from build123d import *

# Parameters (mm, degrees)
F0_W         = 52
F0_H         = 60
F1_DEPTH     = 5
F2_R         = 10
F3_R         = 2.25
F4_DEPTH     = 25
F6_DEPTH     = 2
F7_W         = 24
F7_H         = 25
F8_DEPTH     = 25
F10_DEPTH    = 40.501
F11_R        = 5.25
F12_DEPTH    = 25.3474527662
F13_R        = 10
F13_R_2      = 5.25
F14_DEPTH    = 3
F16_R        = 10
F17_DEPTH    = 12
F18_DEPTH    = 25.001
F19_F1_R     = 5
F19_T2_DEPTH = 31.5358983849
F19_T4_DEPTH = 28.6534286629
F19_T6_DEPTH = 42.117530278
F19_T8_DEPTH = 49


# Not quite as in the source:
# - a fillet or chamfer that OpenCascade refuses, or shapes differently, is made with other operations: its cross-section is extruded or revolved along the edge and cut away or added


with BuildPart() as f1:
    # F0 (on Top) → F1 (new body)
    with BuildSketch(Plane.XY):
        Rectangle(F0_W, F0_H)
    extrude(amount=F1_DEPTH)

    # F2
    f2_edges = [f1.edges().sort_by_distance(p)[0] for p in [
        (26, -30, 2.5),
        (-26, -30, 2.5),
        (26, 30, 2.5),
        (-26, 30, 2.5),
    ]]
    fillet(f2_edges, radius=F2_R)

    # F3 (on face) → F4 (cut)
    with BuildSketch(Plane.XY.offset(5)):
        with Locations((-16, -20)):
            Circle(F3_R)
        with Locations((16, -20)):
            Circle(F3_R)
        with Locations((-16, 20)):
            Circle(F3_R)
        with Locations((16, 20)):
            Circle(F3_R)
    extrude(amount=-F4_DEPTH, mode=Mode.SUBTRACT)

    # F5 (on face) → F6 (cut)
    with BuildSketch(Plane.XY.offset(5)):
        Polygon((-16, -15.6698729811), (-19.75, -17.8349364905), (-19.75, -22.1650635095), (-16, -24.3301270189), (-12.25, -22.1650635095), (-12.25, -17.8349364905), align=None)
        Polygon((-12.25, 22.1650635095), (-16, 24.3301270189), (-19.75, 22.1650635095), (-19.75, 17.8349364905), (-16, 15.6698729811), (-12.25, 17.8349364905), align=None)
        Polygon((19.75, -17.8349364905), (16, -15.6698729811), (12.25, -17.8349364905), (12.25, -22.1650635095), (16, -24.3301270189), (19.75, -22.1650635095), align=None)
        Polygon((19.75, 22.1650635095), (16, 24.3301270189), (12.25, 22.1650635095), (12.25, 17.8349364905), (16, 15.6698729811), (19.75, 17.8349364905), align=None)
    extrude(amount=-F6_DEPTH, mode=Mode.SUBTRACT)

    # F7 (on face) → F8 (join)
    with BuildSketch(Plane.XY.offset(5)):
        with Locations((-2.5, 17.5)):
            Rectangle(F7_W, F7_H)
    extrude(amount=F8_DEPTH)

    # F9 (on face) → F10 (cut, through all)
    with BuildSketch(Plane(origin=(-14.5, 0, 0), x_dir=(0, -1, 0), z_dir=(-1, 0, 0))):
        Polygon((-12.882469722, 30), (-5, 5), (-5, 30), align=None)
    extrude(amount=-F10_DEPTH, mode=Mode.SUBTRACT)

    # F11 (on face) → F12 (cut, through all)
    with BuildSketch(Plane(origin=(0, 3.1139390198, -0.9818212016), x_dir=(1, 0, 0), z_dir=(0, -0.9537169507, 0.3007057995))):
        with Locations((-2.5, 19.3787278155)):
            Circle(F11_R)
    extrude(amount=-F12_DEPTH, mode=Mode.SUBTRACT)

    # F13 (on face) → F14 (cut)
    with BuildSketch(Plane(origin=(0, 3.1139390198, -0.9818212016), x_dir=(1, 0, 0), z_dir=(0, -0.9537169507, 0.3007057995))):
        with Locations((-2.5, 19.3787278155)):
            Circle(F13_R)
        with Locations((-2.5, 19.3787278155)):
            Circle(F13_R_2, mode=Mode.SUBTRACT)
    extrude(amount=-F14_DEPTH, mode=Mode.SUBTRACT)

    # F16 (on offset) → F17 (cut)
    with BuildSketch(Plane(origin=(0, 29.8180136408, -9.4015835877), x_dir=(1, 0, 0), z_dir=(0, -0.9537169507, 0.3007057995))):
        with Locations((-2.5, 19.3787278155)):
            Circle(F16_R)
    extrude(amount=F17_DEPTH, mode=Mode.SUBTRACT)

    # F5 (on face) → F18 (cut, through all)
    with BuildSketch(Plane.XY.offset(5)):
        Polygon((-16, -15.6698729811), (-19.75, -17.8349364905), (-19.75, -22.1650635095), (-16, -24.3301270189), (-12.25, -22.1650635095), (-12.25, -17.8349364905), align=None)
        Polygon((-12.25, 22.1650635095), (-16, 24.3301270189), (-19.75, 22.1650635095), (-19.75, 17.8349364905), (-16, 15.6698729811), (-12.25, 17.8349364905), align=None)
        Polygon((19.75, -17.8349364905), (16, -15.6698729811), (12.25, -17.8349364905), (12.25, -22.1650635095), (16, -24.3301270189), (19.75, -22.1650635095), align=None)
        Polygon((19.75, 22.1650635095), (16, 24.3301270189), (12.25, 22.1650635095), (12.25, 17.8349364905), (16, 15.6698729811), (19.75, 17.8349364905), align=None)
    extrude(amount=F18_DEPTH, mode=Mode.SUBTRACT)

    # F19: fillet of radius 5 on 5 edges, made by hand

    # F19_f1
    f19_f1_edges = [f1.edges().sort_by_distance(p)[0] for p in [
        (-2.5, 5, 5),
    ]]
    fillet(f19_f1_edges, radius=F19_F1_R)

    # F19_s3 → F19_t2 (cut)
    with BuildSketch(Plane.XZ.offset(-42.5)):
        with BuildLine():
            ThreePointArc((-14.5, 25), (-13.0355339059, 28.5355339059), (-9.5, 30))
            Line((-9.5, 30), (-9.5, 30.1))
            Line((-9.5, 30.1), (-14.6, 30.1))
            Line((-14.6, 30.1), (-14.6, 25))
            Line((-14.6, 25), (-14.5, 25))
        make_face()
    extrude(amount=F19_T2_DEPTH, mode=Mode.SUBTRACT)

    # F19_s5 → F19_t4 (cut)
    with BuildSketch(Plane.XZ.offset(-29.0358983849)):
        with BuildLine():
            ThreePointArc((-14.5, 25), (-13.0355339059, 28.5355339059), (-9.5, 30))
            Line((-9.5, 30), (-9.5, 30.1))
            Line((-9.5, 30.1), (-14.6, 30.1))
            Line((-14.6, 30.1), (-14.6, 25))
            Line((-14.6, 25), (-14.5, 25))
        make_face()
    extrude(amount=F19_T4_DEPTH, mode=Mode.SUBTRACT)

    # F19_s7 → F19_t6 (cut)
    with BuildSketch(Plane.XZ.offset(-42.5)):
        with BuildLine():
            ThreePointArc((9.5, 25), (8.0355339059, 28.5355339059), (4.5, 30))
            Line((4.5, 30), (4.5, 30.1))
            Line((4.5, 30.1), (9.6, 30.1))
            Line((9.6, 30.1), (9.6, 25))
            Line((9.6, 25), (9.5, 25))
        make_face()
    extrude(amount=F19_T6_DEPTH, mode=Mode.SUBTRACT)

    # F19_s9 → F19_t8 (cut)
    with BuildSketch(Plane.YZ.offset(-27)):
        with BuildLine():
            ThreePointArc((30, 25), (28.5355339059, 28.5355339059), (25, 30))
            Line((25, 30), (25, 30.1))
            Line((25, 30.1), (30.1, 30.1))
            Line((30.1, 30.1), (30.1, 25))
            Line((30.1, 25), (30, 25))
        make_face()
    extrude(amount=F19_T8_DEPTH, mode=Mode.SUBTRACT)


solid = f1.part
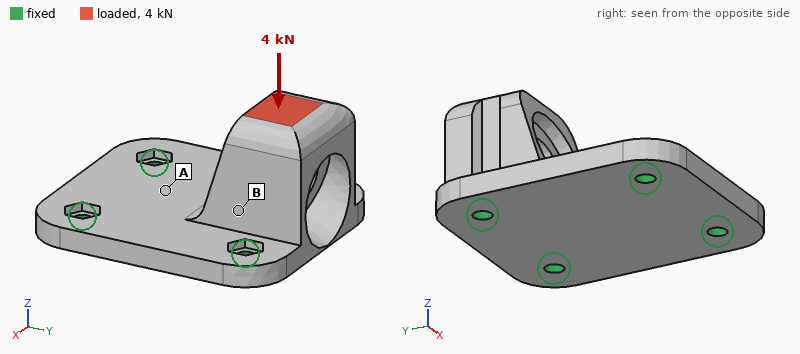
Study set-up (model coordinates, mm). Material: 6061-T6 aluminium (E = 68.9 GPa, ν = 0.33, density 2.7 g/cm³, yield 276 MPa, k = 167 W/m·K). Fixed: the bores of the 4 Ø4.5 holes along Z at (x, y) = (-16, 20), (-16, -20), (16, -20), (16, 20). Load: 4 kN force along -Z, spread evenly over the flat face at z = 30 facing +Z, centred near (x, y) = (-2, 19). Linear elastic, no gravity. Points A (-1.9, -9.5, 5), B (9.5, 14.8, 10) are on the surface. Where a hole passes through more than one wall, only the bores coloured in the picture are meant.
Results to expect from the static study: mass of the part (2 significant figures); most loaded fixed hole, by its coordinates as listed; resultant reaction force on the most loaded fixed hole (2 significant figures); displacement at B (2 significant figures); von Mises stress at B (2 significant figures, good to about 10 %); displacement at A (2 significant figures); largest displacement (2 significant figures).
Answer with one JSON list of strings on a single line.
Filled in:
["61 g", "(-16, 20)", "2.4 kN", "17 µm", "26 MPa", "5.8 µm", "25 µm"]
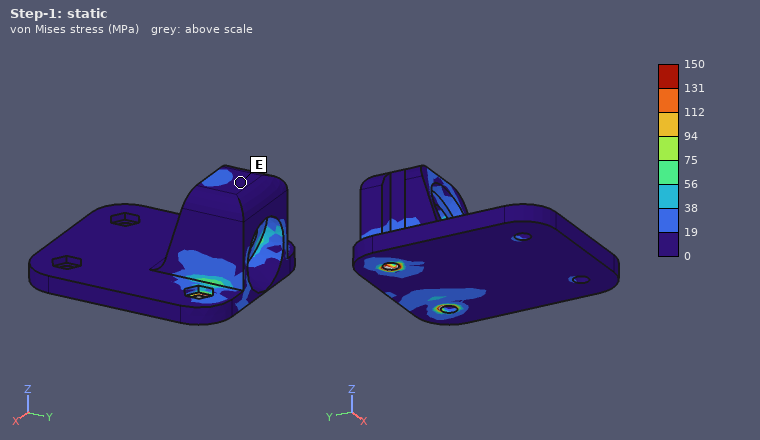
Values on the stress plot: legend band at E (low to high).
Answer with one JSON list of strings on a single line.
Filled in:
["0 to 19 MPa"]
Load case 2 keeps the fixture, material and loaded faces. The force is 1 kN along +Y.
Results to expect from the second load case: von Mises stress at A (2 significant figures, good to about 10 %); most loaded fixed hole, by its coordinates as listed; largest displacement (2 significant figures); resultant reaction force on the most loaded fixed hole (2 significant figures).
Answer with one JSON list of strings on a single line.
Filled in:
["14 MPa", "(-16, -20)", "67 µm", "760 N"]
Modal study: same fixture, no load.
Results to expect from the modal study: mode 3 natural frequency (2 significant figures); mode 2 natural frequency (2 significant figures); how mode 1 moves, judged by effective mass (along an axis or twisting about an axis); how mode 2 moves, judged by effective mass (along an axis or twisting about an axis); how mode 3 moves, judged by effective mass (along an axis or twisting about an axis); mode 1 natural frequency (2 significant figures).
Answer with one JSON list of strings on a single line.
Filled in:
["13 kHz", "9800 Hz", "along Y", "along X", "along Z", "6100 Hz"]
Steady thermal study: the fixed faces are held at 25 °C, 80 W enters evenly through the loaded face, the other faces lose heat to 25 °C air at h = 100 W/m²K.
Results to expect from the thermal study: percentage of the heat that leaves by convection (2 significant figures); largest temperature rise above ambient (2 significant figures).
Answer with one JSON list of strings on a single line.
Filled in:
["19 %", "64 K"]
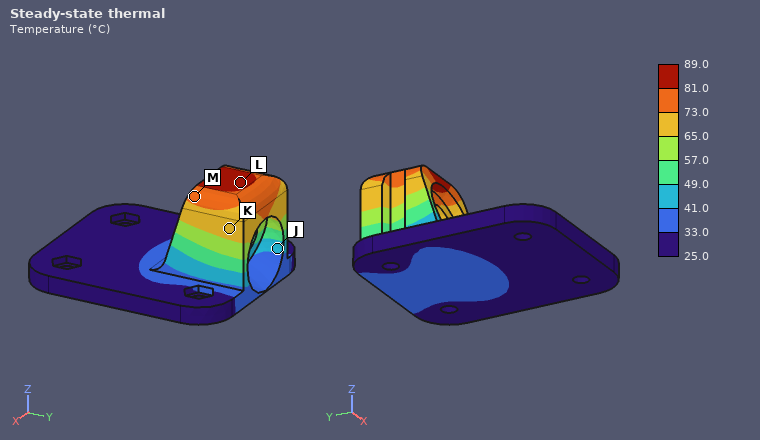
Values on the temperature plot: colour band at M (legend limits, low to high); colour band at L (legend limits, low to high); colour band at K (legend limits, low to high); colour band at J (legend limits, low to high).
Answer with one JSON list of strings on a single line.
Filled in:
["73.0 to 81.0 °C", "81.0 to 89.0 °C", "65.0 to 73.0 °C", "41.0 to 49.0 °C"]
